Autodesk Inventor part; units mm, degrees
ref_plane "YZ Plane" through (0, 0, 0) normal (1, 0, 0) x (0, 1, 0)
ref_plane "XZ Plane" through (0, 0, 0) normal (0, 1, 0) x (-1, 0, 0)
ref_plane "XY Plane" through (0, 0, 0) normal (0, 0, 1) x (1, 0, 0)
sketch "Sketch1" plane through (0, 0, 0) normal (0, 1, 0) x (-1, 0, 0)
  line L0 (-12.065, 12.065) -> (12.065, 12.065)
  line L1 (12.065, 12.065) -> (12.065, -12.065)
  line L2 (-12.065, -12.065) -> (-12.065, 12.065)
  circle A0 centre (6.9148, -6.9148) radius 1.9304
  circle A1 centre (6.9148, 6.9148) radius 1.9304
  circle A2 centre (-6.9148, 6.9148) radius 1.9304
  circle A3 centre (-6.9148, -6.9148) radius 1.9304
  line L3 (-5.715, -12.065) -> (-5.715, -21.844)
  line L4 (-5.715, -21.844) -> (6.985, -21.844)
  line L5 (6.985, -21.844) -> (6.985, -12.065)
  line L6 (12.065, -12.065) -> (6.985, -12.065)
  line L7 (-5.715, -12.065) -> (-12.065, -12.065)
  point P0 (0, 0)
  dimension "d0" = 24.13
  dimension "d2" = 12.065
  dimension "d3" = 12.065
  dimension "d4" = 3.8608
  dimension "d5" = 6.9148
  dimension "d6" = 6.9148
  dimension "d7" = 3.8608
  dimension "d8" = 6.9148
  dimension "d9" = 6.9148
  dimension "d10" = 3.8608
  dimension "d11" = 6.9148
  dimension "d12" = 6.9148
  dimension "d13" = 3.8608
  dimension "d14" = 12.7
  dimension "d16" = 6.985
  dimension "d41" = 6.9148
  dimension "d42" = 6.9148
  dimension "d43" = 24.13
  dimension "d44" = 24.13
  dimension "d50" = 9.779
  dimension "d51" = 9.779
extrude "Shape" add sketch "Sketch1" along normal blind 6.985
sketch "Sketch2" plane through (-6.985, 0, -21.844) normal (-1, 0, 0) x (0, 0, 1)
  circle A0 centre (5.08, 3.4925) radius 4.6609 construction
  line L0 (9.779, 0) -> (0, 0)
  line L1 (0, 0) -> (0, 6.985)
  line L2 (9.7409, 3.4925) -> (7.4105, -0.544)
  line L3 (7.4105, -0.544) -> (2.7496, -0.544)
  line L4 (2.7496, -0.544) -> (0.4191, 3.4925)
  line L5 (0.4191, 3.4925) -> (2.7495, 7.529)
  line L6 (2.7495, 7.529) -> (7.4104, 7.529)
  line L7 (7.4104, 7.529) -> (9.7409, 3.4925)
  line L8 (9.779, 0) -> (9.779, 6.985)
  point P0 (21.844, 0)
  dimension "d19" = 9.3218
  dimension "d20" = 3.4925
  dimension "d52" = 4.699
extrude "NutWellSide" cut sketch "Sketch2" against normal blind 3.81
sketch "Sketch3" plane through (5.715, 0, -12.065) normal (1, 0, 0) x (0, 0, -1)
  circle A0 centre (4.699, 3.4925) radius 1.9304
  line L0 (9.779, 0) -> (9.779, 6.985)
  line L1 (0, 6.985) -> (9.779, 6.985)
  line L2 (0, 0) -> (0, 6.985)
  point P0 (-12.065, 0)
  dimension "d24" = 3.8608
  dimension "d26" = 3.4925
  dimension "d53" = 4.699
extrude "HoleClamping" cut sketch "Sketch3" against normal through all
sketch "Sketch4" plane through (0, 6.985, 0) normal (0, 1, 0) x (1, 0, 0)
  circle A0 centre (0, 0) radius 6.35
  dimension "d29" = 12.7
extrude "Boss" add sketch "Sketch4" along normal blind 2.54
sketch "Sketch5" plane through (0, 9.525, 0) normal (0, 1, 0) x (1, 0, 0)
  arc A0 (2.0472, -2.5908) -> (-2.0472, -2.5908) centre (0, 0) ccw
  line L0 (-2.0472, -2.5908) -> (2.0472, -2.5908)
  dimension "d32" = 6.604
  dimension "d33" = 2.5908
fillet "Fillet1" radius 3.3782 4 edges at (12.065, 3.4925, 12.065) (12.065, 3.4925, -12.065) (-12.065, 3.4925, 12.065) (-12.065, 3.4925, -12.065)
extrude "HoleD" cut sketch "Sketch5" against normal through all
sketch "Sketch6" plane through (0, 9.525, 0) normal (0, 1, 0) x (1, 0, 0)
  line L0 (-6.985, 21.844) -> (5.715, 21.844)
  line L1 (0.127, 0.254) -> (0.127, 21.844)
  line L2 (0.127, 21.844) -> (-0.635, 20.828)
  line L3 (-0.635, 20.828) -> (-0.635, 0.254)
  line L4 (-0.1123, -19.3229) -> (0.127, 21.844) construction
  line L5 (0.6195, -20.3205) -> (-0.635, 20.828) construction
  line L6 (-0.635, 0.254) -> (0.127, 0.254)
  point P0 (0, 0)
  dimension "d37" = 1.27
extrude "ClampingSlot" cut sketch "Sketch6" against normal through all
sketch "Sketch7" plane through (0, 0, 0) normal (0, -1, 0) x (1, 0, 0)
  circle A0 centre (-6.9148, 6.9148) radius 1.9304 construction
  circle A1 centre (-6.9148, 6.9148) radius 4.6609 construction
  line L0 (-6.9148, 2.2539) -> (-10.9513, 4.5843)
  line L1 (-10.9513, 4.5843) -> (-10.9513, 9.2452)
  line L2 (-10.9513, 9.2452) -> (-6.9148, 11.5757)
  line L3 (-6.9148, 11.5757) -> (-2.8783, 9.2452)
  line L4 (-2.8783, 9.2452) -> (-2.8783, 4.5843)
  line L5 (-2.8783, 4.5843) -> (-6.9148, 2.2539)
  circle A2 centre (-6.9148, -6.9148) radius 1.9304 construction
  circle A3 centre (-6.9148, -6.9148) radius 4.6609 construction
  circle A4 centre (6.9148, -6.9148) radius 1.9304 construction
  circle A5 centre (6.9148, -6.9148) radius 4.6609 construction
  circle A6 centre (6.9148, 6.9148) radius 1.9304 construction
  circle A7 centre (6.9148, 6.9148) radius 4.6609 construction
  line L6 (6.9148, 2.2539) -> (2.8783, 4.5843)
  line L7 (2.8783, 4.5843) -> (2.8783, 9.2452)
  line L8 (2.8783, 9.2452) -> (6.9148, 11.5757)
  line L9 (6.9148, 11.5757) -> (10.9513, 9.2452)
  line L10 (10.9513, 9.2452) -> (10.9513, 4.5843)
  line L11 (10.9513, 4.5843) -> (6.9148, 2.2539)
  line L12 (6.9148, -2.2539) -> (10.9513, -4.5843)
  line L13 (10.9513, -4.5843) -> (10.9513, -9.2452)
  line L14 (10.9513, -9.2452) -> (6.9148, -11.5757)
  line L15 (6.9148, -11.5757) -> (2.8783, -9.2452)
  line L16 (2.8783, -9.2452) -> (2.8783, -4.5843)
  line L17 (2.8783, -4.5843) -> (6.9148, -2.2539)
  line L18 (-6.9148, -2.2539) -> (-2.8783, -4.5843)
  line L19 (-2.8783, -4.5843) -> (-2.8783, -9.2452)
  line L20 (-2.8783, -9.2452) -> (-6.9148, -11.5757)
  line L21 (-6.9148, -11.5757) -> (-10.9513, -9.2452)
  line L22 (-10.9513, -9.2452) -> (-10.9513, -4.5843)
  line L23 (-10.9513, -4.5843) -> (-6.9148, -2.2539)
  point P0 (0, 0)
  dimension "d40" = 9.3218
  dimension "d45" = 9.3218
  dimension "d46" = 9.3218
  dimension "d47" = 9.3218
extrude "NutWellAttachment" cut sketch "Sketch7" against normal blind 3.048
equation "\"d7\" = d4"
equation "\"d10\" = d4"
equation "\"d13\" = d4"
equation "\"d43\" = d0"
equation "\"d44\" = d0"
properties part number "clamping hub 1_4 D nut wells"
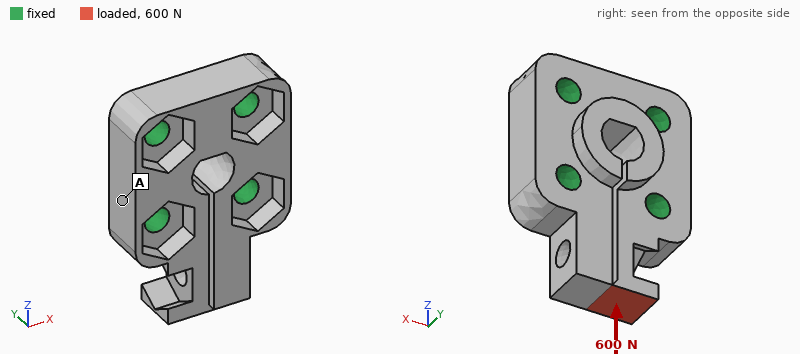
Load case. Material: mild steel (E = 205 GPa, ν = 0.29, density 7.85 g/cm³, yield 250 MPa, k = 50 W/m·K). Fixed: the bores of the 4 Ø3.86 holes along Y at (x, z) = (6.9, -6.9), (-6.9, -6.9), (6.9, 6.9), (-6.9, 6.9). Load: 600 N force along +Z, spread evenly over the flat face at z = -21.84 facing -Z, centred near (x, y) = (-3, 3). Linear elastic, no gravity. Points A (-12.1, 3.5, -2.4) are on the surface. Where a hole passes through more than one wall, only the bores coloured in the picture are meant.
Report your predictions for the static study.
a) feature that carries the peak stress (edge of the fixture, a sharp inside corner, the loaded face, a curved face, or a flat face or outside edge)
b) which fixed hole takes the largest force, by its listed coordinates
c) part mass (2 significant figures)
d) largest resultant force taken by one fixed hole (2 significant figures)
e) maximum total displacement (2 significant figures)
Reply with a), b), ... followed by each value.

a) a curved face
b) (-6.9, -6.9)
c) 28 g
d) 570 N
e) 26 µm
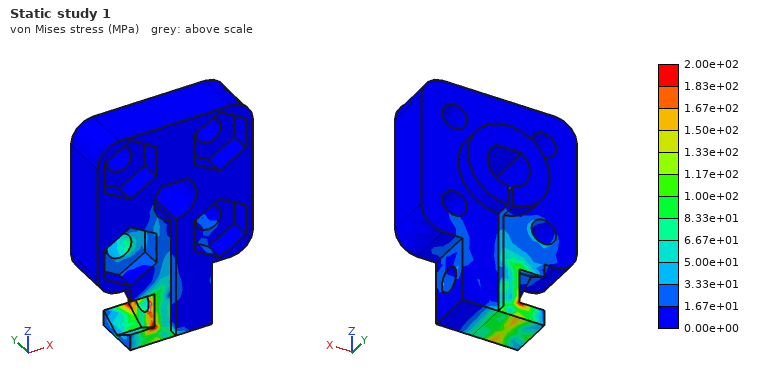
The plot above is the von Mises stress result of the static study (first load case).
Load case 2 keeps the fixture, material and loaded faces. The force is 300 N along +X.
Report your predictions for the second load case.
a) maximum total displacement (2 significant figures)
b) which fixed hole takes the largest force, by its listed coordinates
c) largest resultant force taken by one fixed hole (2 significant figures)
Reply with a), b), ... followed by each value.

a) 14 µm
b) (6.9, -6.9)
c) 350 N
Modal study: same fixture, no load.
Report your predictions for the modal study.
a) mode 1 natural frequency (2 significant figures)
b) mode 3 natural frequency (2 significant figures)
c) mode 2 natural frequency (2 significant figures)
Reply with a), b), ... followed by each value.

a) 17 kHz
b) 29 kHz
c) 23 kHz
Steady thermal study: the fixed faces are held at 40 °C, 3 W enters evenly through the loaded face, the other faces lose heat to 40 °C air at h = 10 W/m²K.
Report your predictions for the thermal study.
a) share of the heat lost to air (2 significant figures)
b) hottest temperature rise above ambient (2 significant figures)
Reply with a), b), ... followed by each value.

a) 3.3 %
b) 40 K
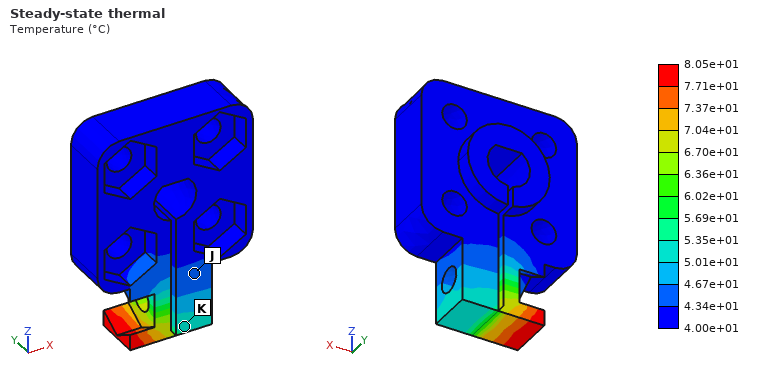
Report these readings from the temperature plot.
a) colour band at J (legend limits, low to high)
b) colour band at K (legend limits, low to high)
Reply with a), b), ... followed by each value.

a) 4.34e+01 to 4.67e+01 °C
b) 5.01e+01 to 5.35e+01 °C
